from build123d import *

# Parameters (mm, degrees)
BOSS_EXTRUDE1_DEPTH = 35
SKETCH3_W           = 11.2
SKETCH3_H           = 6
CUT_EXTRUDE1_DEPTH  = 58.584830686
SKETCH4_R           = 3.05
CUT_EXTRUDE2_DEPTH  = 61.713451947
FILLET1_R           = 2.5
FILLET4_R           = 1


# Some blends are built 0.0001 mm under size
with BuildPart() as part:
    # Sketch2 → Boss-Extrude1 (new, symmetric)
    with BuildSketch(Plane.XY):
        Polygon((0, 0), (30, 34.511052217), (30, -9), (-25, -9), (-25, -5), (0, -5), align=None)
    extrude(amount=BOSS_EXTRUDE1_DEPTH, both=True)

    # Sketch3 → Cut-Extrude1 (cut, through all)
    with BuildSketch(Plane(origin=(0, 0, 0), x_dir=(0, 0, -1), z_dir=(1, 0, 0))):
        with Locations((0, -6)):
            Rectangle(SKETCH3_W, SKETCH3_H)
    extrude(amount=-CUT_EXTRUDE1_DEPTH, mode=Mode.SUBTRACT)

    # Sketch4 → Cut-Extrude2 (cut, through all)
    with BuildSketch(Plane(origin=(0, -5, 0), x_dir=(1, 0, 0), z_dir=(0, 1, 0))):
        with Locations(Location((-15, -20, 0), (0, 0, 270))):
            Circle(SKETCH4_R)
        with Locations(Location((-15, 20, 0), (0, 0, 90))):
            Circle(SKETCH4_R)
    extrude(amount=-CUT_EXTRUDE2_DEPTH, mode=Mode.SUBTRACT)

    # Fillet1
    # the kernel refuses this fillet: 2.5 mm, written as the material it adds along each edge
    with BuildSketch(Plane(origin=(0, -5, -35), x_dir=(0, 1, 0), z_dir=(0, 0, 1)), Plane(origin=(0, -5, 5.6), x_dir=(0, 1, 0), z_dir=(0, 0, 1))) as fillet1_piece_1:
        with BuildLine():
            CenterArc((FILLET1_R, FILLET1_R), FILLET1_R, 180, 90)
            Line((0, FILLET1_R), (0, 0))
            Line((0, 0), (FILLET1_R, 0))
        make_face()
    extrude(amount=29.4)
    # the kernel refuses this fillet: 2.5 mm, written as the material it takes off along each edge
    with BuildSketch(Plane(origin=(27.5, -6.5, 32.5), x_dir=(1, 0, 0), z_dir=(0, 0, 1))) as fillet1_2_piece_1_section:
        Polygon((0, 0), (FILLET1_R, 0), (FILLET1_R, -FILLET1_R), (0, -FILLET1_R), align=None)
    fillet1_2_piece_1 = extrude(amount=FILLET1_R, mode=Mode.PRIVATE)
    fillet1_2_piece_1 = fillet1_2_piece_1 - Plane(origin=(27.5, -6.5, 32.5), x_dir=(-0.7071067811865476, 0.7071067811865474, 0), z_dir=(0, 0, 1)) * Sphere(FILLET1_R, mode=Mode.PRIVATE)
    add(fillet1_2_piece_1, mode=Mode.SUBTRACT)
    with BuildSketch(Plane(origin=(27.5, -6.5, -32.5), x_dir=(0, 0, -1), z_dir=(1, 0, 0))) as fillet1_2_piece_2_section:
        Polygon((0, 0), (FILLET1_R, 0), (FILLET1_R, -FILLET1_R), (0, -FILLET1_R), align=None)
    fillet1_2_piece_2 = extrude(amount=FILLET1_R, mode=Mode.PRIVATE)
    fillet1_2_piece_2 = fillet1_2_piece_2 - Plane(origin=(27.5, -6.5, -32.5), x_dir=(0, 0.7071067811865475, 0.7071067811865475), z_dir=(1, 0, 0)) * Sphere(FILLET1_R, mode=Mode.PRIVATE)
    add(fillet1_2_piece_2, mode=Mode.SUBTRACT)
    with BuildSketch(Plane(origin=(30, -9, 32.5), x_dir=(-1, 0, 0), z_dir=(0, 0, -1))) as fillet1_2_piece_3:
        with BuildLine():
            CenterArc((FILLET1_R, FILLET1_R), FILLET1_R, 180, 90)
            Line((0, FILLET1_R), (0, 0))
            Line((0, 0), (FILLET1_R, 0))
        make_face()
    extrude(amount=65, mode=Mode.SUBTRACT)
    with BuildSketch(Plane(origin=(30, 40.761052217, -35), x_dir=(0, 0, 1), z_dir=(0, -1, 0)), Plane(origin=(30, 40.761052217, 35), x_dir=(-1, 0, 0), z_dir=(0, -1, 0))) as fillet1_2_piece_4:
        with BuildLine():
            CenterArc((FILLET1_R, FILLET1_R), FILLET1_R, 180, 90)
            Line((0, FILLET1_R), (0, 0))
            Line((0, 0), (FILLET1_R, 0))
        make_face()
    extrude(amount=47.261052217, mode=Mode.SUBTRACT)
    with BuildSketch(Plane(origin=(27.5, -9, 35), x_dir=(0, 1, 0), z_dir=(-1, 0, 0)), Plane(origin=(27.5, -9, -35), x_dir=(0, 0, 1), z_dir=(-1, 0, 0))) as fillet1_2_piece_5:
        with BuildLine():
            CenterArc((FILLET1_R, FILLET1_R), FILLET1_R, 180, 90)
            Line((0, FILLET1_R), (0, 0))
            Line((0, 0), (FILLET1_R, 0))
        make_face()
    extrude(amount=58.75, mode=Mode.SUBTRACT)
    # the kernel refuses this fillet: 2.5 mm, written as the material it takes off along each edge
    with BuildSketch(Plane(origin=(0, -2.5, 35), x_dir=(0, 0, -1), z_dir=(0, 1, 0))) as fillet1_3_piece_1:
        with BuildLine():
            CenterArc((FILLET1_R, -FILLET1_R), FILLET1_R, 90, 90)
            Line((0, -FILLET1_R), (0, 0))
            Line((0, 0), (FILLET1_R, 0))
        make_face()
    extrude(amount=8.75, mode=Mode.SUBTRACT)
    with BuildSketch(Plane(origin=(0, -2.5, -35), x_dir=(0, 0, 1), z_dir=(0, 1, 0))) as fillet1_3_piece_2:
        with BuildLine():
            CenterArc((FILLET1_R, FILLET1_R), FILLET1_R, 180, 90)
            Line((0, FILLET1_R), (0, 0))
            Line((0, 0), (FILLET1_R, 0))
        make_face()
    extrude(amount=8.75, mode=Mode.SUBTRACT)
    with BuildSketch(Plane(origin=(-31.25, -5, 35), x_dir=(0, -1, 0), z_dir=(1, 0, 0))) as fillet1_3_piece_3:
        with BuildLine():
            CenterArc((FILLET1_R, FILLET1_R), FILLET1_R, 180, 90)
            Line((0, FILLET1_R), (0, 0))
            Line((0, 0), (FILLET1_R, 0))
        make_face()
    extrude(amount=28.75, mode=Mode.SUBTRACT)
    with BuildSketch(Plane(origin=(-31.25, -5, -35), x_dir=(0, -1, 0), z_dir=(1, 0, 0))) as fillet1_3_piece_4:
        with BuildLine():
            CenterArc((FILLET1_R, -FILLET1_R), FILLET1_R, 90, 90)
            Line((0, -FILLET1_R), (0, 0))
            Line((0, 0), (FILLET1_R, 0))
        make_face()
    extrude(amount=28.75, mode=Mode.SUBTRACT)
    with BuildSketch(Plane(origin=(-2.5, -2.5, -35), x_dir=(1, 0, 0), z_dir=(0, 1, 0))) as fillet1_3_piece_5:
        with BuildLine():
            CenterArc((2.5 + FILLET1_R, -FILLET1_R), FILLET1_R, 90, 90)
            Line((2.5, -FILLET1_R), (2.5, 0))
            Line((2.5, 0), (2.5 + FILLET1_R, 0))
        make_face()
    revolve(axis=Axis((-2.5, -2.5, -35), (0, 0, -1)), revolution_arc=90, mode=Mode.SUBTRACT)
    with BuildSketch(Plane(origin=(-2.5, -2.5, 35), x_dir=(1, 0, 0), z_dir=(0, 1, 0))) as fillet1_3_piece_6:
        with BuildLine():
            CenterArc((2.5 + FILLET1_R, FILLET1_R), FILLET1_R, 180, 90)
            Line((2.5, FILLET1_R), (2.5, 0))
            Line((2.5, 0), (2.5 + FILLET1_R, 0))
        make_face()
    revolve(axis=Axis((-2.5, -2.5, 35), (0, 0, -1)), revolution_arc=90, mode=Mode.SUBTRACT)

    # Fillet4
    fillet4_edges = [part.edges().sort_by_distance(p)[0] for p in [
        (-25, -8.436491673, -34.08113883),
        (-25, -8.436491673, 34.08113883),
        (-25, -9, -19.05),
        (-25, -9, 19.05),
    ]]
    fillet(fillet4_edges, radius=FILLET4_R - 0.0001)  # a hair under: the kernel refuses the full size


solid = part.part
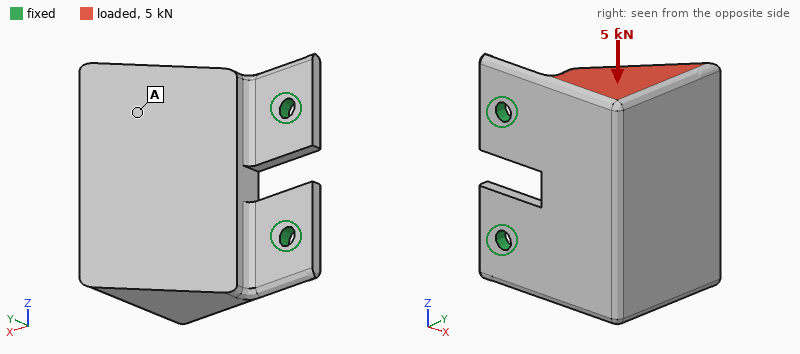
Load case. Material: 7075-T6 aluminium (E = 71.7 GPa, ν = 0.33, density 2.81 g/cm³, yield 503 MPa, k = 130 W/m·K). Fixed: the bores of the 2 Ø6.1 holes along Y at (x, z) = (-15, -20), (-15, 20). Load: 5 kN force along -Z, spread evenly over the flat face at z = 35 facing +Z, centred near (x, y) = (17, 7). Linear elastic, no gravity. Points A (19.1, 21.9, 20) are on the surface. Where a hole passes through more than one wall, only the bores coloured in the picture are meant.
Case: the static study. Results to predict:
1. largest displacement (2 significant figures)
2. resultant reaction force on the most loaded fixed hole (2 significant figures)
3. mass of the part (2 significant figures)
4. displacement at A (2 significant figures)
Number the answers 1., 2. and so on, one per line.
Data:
1. 0.19 mm
2. 4.5 kN
3. 170 g
4. 0.13 mm
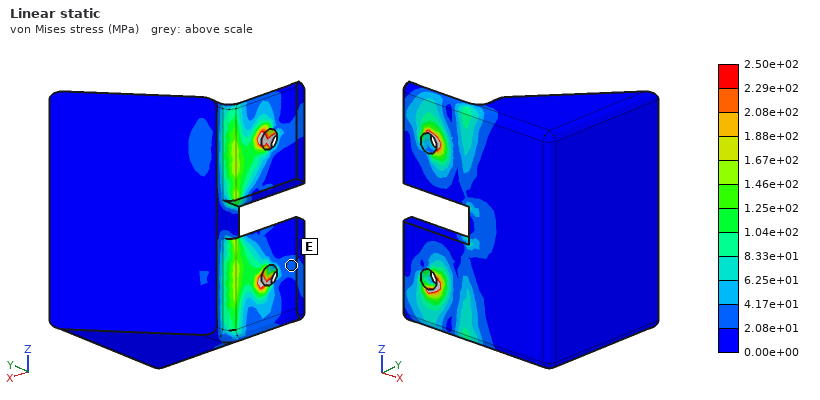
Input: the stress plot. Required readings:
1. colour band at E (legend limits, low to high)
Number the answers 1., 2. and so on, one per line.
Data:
1. 2.08e+01 to 4.17e+01 MPa
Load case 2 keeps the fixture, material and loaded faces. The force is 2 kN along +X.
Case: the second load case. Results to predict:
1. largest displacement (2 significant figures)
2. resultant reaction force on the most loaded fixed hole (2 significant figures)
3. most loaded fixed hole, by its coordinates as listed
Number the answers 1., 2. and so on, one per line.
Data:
1. 1.1 mm
2. 2.6 kN
3. (-15, 20)
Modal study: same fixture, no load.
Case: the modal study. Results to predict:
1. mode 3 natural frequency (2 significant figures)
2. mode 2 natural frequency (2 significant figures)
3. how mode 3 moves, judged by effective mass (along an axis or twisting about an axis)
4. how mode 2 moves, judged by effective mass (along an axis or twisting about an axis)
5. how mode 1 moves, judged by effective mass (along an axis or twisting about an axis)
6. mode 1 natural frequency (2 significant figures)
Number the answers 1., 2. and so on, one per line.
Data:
1. 4500 Hz
2. 2200 Hz
3. along Z
4. along Z
5. along Y
6. 500 Hz
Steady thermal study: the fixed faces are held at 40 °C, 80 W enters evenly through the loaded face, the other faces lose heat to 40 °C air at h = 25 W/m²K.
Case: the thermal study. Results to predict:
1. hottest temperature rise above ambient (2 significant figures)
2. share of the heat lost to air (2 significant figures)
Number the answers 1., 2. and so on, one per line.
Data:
1. 69 K
2. 16 %
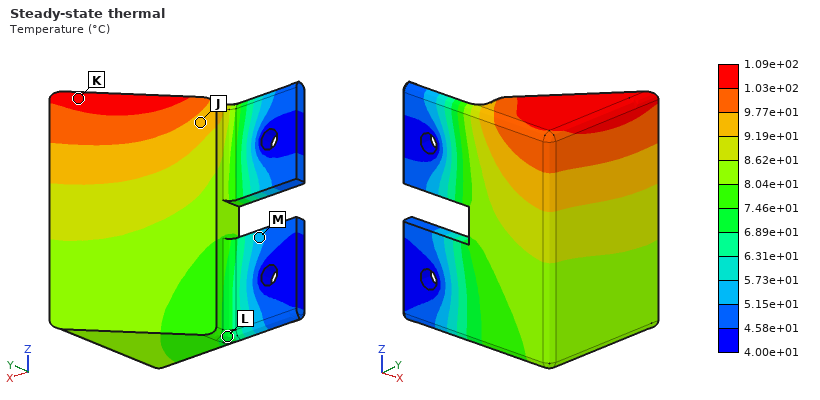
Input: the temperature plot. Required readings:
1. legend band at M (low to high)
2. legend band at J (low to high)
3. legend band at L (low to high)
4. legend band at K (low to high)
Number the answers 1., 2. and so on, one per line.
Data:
1. 5.15e+01 to 5.73e+01 °C
2. 9.19e+01 to 9.77e+01 °C
3. 6.89e+01 to 7.46e+01 °C
4. 1.03e+02 to 1.09e+02 °C
